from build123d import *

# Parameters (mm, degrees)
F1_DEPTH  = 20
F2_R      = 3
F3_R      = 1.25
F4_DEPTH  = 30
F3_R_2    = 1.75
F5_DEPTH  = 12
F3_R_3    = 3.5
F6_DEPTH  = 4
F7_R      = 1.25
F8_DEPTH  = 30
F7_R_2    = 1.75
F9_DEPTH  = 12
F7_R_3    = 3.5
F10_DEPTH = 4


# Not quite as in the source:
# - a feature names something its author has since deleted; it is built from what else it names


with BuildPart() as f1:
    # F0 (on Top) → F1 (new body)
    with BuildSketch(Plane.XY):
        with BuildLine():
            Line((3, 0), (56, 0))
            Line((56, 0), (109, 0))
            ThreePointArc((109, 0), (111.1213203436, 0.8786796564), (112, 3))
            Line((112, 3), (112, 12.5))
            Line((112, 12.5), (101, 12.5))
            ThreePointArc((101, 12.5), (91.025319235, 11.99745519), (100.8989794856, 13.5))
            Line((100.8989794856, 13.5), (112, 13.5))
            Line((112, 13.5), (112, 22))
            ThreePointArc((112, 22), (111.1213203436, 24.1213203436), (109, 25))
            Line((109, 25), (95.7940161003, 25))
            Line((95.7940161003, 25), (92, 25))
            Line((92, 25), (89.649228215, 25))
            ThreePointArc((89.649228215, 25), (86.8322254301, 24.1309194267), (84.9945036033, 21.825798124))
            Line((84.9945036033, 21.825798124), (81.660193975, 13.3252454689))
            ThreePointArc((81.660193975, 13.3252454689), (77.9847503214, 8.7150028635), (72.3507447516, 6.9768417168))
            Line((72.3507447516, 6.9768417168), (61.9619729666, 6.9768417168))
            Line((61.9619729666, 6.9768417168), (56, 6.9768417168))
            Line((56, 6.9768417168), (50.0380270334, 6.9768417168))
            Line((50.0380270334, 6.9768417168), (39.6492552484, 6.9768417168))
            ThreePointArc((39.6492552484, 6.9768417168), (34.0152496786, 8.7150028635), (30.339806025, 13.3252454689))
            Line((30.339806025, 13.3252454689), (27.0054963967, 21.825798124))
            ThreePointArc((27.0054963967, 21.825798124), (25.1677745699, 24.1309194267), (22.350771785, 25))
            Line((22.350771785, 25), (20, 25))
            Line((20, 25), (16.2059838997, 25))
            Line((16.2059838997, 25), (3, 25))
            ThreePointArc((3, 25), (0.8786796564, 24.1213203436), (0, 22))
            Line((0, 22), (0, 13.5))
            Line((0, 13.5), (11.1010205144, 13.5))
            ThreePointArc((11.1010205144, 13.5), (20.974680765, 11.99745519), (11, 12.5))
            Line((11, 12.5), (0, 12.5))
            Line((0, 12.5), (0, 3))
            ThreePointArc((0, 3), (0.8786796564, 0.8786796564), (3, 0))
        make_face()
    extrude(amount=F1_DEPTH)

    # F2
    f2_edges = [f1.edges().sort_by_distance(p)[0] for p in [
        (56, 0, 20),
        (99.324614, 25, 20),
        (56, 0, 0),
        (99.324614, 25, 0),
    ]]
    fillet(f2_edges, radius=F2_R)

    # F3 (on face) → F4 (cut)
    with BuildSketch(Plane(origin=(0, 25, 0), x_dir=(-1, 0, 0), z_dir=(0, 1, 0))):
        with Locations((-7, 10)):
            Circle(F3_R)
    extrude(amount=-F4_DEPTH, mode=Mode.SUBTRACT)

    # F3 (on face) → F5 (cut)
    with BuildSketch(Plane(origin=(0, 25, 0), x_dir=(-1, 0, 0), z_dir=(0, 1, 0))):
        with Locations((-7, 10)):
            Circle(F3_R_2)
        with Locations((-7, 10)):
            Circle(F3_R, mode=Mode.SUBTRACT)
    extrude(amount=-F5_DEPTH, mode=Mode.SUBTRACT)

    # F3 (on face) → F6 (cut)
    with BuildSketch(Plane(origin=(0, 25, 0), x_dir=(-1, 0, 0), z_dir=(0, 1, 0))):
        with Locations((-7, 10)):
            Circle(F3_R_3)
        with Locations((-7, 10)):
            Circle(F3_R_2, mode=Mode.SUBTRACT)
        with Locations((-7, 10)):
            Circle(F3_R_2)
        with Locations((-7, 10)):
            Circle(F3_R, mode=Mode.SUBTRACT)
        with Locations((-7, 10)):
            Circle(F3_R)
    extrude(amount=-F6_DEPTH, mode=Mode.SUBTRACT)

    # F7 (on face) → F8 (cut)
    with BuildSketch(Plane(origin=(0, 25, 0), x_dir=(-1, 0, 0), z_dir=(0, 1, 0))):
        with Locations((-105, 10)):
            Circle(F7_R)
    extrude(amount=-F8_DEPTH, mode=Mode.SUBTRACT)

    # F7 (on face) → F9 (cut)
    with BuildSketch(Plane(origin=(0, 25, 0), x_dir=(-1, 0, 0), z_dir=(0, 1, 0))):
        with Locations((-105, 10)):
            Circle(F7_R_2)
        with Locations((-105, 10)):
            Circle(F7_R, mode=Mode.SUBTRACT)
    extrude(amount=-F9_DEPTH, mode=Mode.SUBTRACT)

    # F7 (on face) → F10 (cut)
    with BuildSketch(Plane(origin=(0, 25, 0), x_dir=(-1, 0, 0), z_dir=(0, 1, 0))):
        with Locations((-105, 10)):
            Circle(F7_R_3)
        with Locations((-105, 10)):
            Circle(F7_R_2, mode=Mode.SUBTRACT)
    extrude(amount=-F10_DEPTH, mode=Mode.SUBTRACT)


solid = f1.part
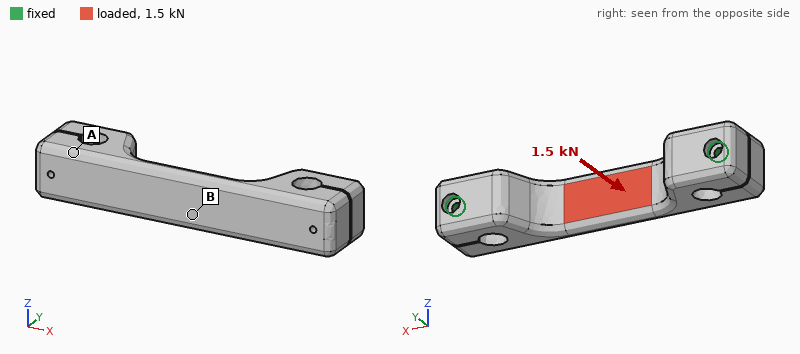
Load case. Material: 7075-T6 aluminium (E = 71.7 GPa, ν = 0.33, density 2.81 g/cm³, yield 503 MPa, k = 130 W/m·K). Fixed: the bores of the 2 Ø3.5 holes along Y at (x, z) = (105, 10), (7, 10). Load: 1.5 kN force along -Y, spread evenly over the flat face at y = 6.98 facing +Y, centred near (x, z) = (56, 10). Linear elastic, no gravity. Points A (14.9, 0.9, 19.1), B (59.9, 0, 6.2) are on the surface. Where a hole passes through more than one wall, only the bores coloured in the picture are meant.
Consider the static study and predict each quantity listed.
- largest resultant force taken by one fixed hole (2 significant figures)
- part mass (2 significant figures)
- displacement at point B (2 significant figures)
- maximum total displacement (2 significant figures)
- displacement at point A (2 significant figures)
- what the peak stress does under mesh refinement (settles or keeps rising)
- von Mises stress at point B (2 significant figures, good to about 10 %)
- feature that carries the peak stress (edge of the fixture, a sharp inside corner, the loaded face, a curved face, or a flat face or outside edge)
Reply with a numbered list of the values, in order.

1. 1.4 kN
2. 89 g
3. 43 µm
4. 46 µm
5. 12 µm
6. keeps rising
7. 38 MPa
8. edge of the fixture
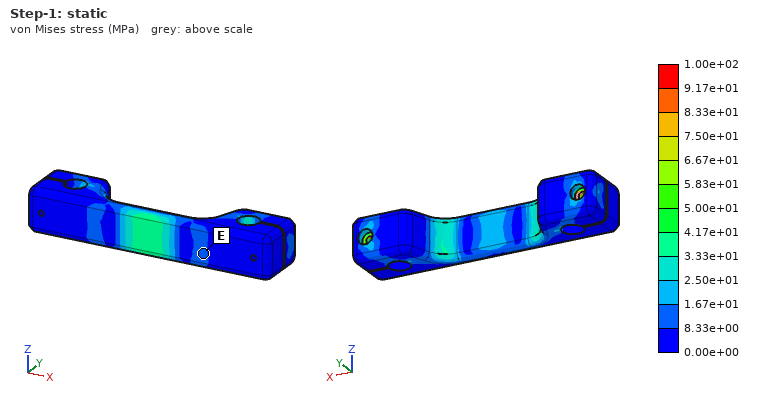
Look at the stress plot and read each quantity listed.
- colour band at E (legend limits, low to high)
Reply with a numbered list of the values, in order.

1. 8.33e+00 to 1.67e+01 MPa
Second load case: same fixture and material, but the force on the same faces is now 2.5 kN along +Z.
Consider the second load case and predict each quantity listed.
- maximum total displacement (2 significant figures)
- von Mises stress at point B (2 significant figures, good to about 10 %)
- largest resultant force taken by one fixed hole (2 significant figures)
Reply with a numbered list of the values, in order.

1. 0.18 mm
2. 33 MPa
3. 1.3 kN
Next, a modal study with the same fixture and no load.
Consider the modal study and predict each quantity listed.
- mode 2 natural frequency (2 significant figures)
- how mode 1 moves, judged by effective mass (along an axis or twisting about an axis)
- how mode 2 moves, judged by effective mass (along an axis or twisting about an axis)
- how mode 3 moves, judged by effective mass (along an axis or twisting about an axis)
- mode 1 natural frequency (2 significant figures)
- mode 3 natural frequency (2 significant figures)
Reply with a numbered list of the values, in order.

1. 4600 Hz
2. along Z
3. twisting about Y
4. along Y
5. 3000 Hz
6. 5500 Hz
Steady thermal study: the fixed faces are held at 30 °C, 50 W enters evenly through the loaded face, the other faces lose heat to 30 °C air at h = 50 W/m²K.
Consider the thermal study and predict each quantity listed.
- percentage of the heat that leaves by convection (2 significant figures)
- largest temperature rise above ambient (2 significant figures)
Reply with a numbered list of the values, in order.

1. 23 %
2. 54 K
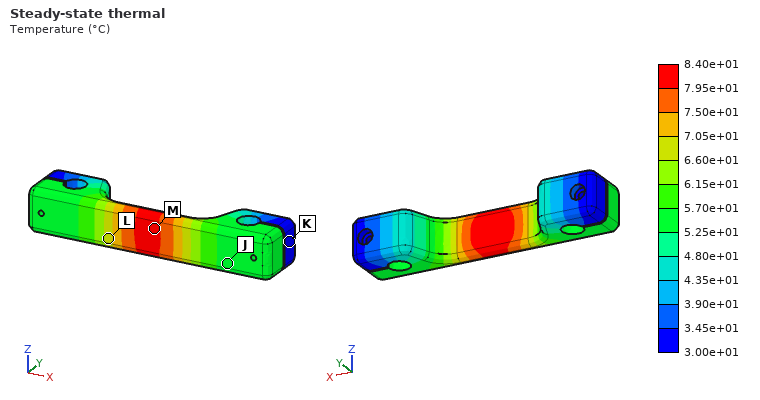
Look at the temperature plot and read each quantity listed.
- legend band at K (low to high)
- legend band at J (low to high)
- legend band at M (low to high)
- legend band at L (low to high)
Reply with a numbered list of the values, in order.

1. 3.00e+01 to 3.45e+01 °C
2. 5.25e+01 to 5.70e+01 °C
3. 7.95e+01 to 8.40e+01 °C
4. 6.60e+01 to 7.05e+01 °C
